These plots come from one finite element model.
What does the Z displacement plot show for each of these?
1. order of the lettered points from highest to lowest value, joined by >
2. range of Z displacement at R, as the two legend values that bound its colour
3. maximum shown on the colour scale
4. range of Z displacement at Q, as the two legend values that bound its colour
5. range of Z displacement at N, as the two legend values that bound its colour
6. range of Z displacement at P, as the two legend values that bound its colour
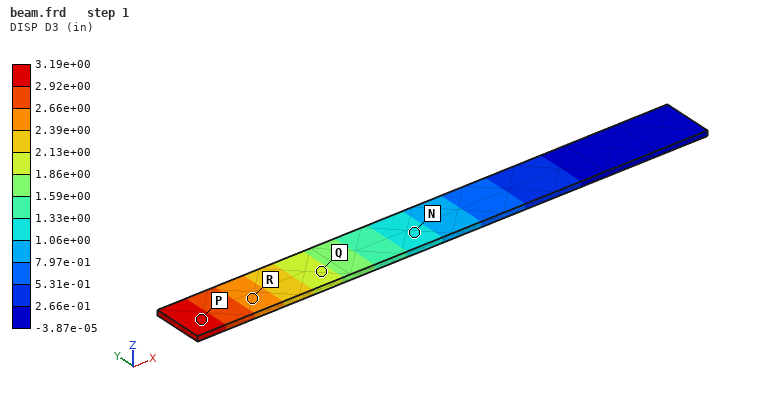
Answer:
P > R > Q > N
2.39e+00 to 2.66e+00 in
3.19e+00 in
1.86e+00 to 2.13e+00 in
1.06e+00 to 1.33e+00 in
2.92e+00 to 3.19e+00 in
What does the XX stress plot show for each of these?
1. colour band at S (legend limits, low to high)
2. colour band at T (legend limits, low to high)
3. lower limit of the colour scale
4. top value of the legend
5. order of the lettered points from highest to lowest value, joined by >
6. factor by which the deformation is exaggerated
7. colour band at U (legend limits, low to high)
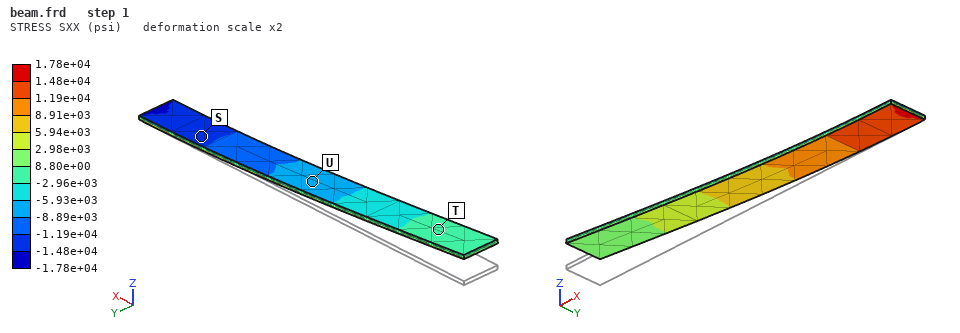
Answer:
-1.48e+04 to -1.19e+04 psi
-2.96e+03 to 8.80e+00 psi
-1.78e+04 psi
1.78e+04 psi
T > U > S
2
-8.89e+03 to -5.93e+03 psi
